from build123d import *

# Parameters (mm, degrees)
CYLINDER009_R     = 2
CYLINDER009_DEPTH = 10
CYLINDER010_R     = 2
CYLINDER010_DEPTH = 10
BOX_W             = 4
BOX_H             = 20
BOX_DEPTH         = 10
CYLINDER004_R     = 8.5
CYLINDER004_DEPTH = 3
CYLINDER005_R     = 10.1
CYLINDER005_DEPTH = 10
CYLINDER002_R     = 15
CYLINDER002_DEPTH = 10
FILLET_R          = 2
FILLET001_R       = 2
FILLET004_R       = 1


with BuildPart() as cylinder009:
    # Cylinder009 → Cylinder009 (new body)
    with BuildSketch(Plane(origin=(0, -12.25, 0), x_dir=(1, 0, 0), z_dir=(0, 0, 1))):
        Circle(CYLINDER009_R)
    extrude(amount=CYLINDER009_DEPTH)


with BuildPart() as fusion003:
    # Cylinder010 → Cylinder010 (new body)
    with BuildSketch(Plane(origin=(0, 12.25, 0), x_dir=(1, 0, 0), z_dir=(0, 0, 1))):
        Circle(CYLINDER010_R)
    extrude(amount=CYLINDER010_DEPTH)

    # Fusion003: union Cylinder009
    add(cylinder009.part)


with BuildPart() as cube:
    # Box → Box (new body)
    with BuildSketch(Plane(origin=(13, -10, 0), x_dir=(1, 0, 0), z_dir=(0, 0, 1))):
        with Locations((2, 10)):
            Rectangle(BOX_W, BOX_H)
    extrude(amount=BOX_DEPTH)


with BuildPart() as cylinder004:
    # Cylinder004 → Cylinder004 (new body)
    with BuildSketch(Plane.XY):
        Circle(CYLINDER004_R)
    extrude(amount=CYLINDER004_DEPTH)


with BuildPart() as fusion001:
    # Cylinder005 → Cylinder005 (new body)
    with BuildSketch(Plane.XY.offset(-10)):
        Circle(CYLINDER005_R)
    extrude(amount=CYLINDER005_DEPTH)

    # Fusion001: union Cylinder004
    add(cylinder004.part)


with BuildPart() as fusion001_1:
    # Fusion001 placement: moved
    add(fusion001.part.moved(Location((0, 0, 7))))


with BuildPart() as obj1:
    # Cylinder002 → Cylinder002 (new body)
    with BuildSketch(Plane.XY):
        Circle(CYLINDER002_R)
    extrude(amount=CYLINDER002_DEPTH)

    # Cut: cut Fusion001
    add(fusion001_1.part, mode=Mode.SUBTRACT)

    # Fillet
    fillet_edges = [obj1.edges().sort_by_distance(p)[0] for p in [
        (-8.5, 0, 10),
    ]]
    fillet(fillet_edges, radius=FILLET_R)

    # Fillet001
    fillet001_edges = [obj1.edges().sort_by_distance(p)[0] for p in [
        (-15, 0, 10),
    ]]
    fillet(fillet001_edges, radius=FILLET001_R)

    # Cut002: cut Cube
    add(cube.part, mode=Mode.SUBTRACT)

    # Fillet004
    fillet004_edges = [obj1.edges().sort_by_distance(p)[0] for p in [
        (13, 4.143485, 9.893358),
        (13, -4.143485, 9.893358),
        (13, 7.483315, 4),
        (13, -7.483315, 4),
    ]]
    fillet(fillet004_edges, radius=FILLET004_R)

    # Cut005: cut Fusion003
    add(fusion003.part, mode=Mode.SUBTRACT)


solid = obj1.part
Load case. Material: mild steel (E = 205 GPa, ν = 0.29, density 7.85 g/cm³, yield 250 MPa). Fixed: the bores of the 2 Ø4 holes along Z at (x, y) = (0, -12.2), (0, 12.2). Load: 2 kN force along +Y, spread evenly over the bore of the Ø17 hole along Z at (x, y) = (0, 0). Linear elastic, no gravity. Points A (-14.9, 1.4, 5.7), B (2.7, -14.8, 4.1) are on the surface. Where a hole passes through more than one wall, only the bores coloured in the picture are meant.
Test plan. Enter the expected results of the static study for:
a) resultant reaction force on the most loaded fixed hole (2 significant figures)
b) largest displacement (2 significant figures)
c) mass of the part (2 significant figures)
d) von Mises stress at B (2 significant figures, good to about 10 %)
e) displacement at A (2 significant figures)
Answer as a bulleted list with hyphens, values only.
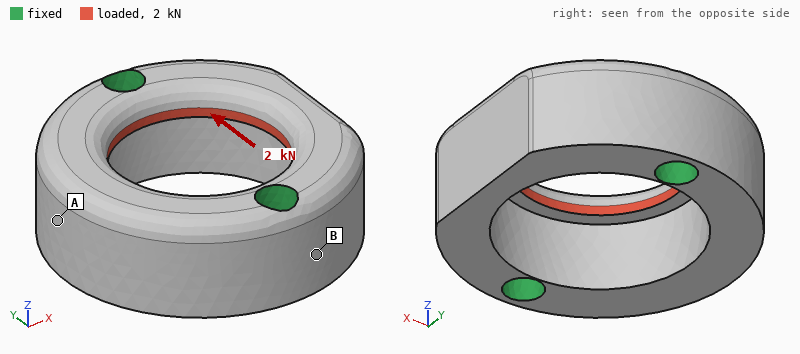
- 1.0 kN
- 2.5 µm
- 28 g
- 18 MPa
- 1.1 µm
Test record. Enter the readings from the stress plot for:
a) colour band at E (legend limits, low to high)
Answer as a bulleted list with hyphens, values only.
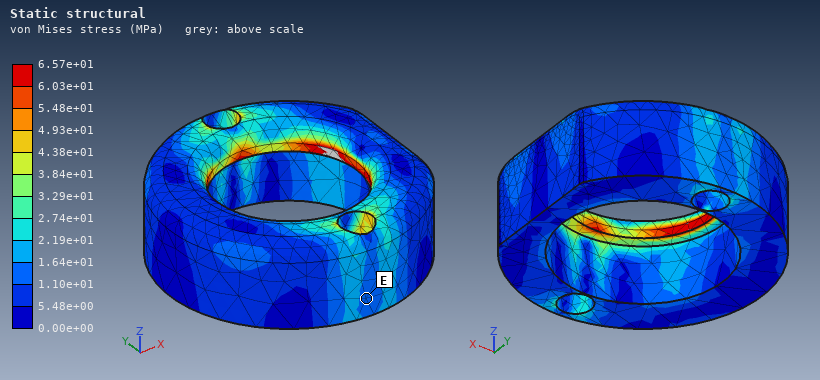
- 1.10e+01 to 1.64e+01 MPa
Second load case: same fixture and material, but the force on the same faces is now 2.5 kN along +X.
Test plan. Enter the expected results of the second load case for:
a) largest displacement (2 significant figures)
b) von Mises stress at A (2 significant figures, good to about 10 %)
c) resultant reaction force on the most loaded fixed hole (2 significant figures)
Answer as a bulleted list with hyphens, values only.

- 2.9 µm
- 13 MPa
- 1.3 kN
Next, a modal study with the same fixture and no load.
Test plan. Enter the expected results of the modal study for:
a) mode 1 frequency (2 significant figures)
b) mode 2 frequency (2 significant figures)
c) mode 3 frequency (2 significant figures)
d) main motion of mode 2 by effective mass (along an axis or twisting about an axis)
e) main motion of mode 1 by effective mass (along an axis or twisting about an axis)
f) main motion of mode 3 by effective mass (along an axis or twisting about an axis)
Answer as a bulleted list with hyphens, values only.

- 25 kHz
- 29 kHz
- 32 kHz
- along Z
- along Z
- along Y
